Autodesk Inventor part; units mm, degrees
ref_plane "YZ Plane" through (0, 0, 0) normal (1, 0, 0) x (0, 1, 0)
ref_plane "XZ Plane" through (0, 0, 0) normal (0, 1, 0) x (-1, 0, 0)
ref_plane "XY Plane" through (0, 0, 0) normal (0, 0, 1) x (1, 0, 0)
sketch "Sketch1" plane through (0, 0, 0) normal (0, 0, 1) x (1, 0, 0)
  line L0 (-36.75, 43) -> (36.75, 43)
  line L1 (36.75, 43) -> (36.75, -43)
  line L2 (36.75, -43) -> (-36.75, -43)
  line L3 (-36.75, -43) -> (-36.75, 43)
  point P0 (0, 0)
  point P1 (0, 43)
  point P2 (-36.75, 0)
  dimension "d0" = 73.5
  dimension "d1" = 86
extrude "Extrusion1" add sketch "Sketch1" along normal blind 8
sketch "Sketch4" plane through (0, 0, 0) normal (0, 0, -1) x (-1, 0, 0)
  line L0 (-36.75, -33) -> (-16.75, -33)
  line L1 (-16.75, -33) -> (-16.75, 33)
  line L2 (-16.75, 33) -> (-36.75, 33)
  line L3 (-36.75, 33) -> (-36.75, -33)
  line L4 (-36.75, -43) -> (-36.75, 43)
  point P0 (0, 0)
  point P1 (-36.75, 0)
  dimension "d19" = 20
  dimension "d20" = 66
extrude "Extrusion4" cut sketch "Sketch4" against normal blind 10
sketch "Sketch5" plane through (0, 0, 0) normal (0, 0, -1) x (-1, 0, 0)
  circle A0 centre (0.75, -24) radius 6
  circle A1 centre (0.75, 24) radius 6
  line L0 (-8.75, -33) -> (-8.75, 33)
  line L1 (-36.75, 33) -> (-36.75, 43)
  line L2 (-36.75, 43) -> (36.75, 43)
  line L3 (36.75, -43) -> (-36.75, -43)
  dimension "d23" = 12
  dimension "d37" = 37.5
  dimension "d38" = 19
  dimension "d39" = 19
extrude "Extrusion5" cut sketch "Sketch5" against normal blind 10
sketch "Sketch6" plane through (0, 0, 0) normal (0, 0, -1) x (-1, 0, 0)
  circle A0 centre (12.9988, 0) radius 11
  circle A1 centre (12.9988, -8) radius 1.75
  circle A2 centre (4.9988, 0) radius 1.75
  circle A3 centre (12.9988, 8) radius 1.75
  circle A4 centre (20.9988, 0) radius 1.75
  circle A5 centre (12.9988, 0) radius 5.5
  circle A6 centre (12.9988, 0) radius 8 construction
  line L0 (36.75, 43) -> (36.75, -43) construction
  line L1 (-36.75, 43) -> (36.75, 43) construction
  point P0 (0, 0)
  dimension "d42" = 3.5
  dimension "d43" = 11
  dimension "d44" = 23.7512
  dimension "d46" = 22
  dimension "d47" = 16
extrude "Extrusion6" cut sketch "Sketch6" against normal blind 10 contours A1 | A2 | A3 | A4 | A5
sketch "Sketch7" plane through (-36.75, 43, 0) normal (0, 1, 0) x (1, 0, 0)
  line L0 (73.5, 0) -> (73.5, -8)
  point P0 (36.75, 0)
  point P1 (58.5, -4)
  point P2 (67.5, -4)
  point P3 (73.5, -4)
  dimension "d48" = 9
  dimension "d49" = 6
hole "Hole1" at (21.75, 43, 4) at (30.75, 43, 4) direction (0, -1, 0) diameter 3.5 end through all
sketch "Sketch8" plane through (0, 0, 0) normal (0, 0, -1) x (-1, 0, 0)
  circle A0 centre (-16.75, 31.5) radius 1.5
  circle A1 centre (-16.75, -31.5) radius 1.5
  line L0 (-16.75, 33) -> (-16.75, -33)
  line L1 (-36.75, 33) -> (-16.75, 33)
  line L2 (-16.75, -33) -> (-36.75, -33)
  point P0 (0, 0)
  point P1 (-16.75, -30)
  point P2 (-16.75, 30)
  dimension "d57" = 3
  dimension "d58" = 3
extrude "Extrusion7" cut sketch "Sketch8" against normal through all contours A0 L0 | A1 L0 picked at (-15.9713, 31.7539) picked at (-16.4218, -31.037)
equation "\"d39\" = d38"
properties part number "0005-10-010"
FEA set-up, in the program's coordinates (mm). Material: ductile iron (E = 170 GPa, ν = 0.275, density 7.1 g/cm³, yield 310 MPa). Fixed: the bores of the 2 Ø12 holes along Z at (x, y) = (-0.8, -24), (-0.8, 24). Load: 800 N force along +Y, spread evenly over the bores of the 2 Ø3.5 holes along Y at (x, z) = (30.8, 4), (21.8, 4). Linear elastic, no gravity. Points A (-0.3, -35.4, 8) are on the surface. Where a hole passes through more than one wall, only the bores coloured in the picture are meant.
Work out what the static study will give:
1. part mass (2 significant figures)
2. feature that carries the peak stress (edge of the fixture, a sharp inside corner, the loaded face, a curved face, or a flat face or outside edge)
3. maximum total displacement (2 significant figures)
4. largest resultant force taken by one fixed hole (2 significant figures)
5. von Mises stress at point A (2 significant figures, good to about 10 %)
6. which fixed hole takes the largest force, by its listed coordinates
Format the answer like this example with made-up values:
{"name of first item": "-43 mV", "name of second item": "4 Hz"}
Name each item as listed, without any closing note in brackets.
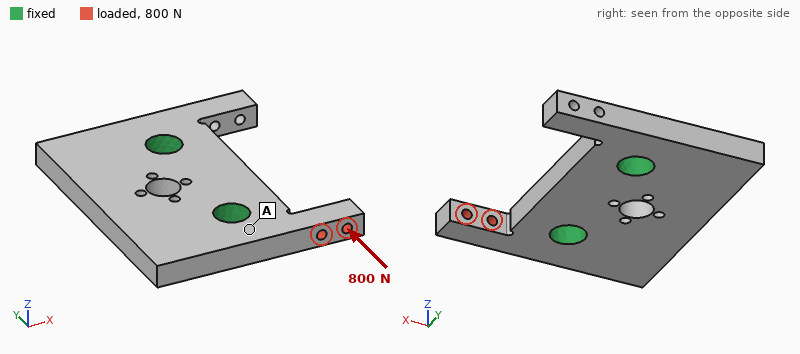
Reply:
{"part mass": "260 g", "feature that carries the peak stress": "a curved face", "maximum total displacement": "28 µm", "largest resultant force taken by one fixed hole": "760 N", "von Mises stress at point A": "11 MPa", "which fixed hole takes the largest force, by its listed coordinates": "(-0.8, -24)"}
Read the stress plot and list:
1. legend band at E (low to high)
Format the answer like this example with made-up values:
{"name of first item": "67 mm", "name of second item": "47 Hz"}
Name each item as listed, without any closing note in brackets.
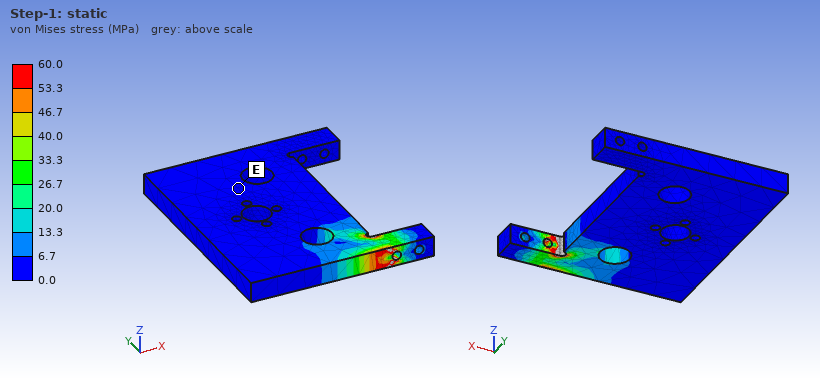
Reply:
{"legend band at E": "0.0 to 6.7 MPa"}
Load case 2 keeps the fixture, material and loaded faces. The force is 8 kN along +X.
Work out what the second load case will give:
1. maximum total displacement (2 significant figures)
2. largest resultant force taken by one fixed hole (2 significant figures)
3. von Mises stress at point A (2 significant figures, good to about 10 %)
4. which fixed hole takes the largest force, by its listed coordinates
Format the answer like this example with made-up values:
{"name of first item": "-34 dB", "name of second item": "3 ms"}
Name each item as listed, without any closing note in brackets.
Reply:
{"maximum total displacement": "39 µm", "largest resultant force taken by one fixed hole": "9.0 kN", "von Mises stress at point A": "58 MPa", "which fixed hole takes the largest force, by its listed coordinates": "(-0.8, -24)"}
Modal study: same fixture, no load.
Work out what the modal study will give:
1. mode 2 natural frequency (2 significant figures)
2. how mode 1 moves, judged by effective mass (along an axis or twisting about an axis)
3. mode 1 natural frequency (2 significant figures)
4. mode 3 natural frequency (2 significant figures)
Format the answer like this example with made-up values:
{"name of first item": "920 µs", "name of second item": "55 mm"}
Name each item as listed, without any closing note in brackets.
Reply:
{"mode 2 natural frequency": "6000 Hz", "how mode 1 moves, judged by effective mass": "along Z", "mode 1 natural frequency": "5100 Hz", "mode 3 natural frequency": "6100 Hz"}
